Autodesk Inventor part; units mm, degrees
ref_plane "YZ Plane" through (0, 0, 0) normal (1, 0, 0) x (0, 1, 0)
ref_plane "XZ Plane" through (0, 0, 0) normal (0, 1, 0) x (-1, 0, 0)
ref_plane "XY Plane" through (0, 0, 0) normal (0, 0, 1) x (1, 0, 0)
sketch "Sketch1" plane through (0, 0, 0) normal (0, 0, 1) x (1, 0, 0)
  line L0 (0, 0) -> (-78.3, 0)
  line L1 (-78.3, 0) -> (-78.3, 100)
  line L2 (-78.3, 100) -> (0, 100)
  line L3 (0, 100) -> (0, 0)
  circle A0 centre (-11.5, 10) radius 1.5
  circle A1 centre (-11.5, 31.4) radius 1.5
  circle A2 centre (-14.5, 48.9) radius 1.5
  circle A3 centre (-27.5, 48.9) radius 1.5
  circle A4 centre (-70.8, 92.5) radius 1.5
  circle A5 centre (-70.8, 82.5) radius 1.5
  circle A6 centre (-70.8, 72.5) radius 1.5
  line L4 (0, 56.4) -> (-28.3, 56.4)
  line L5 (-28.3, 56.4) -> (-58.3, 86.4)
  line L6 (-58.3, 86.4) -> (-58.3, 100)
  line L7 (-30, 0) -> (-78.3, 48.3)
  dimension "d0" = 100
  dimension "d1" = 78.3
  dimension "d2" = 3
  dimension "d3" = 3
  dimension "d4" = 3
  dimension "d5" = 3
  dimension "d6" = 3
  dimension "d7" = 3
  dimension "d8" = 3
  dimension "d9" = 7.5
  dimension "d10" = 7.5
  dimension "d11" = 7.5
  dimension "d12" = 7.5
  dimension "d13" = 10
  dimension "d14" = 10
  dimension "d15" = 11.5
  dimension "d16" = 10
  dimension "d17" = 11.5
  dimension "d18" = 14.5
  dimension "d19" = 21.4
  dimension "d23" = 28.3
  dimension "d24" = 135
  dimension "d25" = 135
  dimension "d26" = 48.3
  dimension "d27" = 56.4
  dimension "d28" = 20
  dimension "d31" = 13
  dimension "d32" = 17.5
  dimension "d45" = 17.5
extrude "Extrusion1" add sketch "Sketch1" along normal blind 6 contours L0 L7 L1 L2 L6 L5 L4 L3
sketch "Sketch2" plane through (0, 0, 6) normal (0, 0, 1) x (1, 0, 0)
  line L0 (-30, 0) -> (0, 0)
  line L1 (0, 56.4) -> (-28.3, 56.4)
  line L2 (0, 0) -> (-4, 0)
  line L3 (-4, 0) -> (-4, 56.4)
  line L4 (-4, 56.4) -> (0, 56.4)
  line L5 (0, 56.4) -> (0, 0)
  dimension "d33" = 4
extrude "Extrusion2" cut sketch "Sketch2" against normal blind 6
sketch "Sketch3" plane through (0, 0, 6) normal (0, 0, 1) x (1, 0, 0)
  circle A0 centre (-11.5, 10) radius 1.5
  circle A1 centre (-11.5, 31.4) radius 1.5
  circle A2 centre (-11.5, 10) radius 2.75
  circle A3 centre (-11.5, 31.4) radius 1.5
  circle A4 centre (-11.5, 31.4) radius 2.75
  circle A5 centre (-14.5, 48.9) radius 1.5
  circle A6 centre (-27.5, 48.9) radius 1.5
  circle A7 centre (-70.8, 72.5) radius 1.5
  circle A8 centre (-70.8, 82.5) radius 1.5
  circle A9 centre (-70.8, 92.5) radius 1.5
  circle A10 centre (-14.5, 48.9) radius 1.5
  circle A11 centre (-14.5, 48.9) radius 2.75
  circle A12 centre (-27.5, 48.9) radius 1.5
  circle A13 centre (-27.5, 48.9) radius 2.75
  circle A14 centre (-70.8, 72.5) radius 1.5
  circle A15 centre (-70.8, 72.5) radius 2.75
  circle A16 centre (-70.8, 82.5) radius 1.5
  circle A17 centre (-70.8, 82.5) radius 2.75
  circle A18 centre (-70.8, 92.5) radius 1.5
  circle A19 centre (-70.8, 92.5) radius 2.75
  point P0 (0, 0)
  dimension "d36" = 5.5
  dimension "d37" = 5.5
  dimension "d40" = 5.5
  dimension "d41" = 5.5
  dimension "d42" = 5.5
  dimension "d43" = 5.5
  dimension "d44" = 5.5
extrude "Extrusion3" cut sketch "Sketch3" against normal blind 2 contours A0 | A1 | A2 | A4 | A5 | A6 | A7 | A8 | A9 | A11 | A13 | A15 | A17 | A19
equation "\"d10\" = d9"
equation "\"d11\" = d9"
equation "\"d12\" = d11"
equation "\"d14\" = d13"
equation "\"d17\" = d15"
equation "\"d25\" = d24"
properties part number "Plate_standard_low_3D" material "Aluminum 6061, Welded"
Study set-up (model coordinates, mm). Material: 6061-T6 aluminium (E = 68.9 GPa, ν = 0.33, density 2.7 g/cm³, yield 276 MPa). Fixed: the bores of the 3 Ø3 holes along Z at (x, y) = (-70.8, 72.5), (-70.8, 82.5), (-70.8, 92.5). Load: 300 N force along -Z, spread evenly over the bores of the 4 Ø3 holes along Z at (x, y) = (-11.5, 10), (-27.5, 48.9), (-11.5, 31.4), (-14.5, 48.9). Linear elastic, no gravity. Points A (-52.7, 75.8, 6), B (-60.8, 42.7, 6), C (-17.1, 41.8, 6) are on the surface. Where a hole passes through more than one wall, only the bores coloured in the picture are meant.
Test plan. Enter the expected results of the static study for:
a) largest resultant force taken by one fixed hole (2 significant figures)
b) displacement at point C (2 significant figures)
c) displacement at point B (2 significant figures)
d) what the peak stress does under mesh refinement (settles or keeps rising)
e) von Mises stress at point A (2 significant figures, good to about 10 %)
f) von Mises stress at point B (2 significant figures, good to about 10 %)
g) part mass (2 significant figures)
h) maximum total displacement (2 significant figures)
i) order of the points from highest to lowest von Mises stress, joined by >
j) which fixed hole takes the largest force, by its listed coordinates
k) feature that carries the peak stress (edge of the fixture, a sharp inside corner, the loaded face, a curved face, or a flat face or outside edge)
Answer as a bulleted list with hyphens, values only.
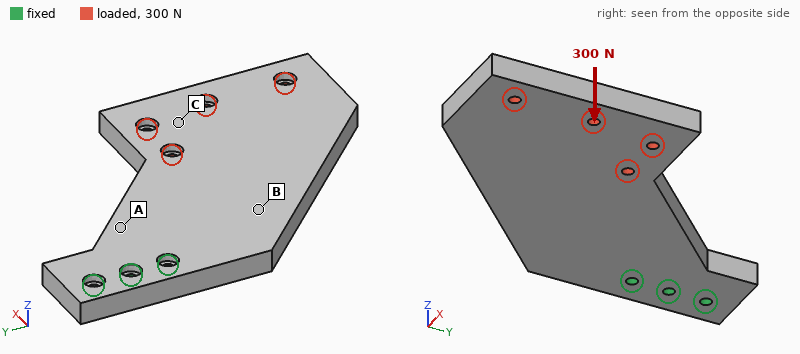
- 860 N
- 0.80 mm
- 0.22 mm
- keeps rising
- 82 MPa
- 43 MPa
- 69 g
- 1.4 mm
- A > B > C
- (-70.8, 72.5)
- edge of the fixture
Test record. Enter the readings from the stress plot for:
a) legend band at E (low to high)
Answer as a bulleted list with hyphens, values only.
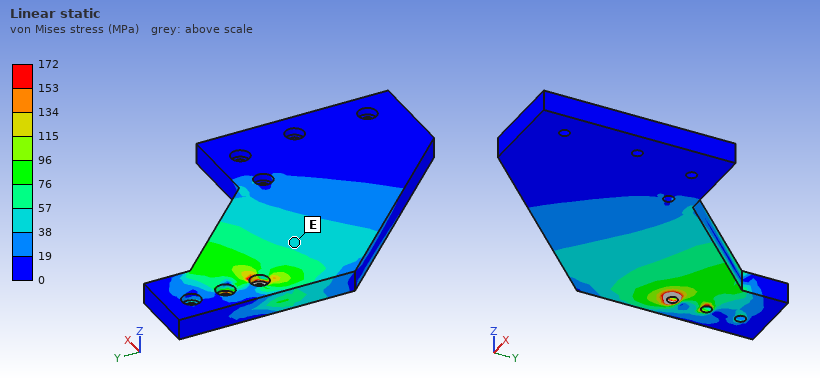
- 38 to 57 MPa
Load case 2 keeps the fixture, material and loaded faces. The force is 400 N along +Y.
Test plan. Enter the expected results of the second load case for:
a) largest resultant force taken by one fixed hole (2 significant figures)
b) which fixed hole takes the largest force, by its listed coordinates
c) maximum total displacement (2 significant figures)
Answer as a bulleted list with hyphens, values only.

- 1.2 kN
- (-70.8, 72.5)
- 0.10 mm
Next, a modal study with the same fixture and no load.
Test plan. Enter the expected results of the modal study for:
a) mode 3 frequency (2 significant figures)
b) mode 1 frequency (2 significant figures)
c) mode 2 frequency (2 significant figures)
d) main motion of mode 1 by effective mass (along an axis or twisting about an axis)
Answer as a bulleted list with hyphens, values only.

- 1900 Hz
- 490 Hz
- 1800 Hz
- along Z
